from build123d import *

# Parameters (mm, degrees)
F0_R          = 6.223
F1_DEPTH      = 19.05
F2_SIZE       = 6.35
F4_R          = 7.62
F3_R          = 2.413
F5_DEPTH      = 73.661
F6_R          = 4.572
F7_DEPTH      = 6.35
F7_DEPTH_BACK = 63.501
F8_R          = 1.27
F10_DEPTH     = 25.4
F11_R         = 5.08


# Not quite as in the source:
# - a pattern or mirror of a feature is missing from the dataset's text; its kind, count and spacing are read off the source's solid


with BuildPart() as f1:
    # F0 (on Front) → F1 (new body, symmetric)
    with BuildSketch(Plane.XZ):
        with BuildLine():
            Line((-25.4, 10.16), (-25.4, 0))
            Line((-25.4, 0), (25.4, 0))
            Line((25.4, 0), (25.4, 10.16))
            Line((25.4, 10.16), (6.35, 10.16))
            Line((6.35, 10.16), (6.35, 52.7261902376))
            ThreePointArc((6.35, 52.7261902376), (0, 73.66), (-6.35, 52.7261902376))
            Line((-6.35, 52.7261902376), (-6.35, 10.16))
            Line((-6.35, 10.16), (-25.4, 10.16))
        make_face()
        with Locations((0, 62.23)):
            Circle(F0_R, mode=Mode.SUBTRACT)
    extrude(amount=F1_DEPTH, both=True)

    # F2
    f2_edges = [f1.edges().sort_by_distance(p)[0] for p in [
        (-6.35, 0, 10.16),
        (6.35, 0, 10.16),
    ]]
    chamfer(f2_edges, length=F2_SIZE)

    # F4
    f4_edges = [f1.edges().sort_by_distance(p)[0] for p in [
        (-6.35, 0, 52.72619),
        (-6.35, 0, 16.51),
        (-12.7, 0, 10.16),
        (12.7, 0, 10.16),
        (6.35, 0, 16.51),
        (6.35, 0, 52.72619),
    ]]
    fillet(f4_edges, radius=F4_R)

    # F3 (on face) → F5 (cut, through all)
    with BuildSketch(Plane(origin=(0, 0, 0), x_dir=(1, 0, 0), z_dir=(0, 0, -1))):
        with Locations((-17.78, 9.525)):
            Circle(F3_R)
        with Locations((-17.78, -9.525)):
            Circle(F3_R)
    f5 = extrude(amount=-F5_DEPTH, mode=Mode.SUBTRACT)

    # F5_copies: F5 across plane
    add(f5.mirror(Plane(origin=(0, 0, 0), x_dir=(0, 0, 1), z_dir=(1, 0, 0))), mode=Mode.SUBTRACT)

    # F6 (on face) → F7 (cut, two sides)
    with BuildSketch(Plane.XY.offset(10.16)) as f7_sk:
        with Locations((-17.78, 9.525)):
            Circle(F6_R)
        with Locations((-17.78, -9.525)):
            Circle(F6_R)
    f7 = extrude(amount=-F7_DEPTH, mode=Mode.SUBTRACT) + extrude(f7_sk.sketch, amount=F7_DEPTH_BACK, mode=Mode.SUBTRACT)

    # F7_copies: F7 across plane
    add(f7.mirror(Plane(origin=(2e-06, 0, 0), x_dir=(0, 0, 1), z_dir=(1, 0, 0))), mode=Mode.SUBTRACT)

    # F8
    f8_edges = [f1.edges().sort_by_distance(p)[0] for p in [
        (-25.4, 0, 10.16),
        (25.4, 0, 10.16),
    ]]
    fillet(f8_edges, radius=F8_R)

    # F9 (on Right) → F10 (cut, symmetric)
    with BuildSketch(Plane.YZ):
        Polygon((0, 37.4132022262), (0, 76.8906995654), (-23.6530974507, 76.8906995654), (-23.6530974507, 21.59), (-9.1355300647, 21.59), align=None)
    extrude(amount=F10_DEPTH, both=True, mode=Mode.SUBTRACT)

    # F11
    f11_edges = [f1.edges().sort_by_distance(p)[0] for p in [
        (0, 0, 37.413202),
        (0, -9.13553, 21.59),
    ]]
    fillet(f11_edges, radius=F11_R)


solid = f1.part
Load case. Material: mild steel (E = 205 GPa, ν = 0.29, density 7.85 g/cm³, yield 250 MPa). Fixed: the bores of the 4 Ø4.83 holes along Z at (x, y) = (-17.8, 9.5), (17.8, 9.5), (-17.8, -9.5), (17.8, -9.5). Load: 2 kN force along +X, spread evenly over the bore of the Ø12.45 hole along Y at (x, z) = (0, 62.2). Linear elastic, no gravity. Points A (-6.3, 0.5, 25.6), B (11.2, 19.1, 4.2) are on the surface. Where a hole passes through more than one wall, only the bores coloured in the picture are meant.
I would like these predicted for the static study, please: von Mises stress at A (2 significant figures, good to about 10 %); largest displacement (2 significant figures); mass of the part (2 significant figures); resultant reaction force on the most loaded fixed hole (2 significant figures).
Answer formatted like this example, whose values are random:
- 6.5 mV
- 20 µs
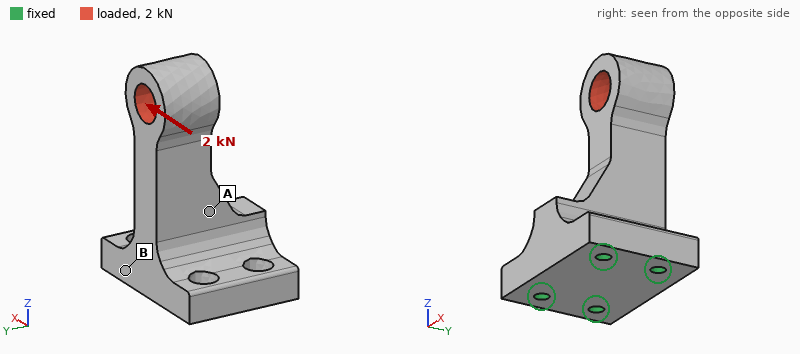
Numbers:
- 110 MPa
- 0.15 mm
- 300 g
- 2.1 kN
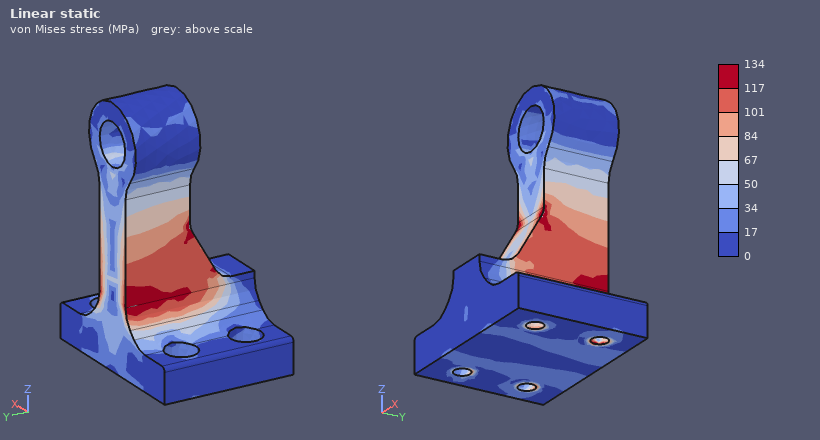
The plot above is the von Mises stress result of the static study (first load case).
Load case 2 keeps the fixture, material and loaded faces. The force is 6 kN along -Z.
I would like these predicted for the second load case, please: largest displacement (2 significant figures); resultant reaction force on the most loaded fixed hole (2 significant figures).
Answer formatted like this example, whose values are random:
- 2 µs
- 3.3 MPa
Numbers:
- 28 µm
- 3.2 kN
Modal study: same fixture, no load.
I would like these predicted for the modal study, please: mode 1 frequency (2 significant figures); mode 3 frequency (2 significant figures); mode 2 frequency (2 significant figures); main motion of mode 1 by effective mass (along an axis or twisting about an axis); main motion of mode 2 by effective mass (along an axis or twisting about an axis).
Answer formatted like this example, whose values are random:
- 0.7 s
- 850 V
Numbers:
- 2900 Hz
- 11 kHz
- 3700 Hz
- along X
- along Y
